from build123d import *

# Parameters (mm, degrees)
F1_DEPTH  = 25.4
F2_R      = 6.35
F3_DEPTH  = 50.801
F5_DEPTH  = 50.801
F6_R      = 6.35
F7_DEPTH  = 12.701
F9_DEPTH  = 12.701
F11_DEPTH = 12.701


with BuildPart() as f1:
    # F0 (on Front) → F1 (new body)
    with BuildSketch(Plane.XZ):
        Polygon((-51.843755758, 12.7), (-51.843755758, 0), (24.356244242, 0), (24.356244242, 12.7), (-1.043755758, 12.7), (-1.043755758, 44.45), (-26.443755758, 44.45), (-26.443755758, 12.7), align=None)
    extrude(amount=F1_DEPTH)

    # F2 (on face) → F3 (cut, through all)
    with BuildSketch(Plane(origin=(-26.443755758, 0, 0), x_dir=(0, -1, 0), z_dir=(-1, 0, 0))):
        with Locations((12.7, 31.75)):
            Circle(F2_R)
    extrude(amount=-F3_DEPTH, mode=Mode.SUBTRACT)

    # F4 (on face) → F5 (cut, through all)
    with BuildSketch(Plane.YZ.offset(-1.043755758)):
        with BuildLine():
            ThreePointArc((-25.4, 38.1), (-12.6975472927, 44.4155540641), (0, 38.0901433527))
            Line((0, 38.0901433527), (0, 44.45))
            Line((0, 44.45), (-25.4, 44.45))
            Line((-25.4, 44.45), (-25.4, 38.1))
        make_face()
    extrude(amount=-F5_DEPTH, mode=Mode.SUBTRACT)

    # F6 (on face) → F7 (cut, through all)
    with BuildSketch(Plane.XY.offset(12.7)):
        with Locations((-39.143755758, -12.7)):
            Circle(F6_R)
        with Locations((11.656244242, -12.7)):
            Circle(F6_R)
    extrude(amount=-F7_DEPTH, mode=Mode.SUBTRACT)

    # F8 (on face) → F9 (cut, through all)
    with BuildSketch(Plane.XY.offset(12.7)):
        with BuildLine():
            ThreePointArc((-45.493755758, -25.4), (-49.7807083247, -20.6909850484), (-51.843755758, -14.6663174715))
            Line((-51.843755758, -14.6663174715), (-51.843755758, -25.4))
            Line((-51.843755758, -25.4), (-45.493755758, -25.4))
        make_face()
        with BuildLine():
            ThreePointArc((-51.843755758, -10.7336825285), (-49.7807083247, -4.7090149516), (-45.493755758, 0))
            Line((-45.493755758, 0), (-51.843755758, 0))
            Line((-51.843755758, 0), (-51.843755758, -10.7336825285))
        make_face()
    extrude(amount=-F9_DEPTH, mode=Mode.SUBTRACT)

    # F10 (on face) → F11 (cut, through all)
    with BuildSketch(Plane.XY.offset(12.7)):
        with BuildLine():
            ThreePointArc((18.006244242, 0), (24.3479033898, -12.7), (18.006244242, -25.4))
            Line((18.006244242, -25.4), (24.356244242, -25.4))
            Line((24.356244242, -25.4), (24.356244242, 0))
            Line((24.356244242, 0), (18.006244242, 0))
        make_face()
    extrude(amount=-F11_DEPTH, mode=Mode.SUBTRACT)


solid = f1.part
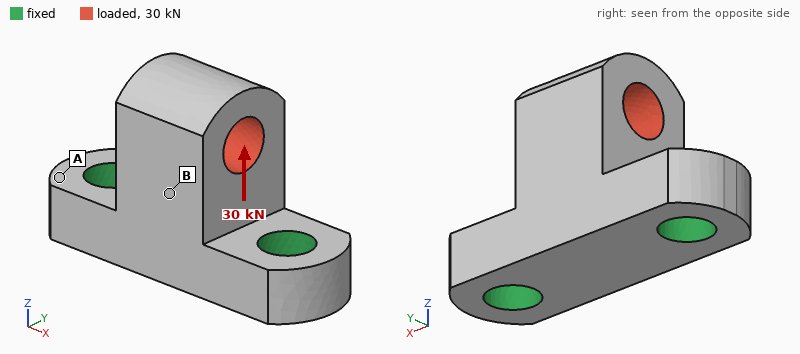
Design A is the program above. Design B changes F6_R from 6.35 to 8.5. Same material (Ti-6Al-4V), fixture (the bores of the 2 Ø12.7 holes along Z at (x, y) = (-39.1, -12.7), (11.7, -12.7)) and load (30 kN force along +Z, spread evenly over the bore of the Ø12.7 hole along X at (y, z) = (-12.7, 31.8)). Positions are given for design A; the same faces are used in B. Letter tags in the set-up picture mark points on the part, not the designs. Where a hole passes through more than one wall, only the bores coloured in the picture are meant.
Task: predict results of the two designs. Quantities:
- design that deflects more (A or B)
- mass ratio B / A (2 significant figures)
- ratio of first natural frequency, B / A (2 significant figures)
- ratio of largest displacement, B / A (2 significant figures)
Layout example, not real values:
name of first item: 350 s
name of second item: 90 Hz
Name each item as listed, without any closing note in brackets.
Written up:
design that deflects more: A
mass ratio B / A: 0.93
ratio of first natural frequency, B / A: 1.1
ratio of largest displacement, B / A: 0.85
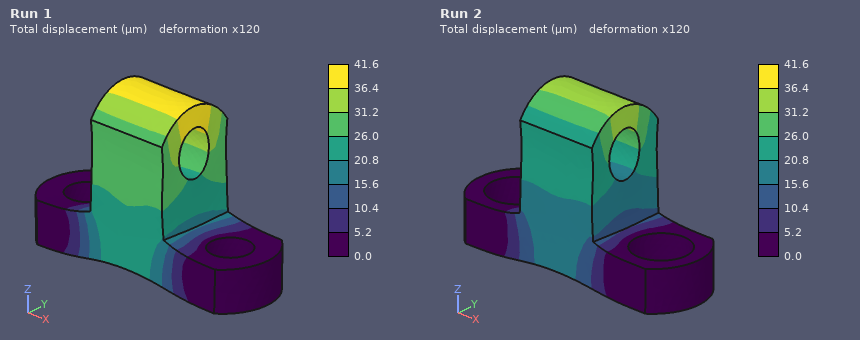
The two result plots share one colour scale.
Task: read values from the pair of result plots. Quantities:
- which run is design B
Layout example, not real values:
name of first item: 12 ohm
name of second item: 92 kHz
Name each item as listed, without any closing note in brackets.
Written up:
which run is design B: Run 2
